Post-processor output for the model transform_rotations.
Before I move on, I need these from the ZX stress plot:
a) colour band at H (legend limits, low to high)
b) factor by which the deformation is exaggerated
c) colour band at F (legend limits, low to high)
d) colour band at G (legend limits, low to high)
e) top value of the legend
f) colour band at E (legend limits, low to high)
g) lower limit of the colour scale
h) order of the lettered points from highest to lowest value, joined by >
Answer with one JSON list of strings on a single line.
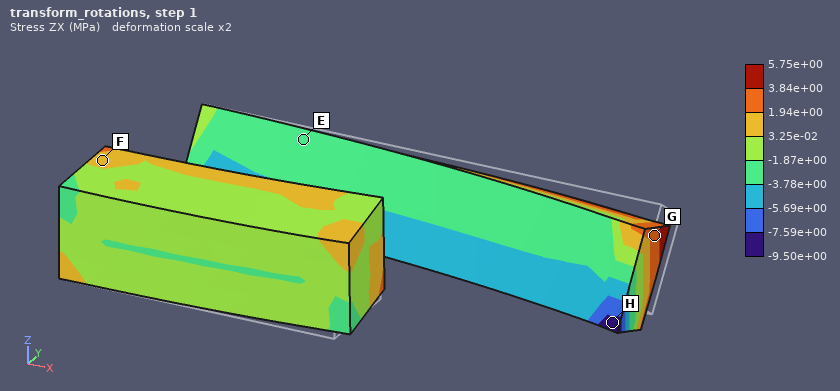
["-9.50e+00 to -7.59e+00 MPa", "2", "3.25e-02 to 1.94e+00 MPa", "1.94e+00 to 3.84e+00 MPa", "5.75e+00 MPa", "-3.78e+00 to -1.87e+00 MPa", "-9.50e+00 MPa", "G > F > E > H"]
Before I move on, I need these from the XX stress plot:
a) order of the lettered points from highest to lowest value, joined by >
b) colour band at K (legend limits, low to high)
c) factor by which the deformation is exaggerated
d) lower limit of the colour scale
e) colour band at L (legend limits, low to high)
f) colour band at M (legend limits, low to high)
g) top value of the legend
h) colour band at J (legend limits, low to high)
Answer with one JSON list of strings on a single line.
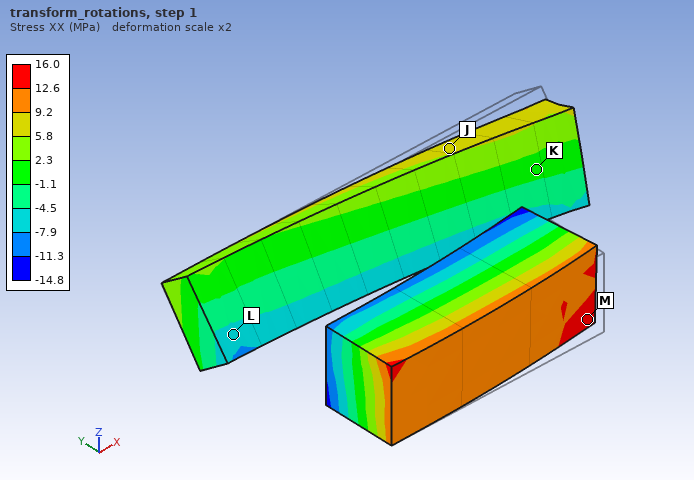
["M > J > K > L", "-1.1 to 2.3 MPa", "2", "-14.8 MPa", "-7.9 to -4.5 MPa", "12.6 to 16.0 MPa", "16.0 MPa", "5.8 to 9.2 MPa"]
